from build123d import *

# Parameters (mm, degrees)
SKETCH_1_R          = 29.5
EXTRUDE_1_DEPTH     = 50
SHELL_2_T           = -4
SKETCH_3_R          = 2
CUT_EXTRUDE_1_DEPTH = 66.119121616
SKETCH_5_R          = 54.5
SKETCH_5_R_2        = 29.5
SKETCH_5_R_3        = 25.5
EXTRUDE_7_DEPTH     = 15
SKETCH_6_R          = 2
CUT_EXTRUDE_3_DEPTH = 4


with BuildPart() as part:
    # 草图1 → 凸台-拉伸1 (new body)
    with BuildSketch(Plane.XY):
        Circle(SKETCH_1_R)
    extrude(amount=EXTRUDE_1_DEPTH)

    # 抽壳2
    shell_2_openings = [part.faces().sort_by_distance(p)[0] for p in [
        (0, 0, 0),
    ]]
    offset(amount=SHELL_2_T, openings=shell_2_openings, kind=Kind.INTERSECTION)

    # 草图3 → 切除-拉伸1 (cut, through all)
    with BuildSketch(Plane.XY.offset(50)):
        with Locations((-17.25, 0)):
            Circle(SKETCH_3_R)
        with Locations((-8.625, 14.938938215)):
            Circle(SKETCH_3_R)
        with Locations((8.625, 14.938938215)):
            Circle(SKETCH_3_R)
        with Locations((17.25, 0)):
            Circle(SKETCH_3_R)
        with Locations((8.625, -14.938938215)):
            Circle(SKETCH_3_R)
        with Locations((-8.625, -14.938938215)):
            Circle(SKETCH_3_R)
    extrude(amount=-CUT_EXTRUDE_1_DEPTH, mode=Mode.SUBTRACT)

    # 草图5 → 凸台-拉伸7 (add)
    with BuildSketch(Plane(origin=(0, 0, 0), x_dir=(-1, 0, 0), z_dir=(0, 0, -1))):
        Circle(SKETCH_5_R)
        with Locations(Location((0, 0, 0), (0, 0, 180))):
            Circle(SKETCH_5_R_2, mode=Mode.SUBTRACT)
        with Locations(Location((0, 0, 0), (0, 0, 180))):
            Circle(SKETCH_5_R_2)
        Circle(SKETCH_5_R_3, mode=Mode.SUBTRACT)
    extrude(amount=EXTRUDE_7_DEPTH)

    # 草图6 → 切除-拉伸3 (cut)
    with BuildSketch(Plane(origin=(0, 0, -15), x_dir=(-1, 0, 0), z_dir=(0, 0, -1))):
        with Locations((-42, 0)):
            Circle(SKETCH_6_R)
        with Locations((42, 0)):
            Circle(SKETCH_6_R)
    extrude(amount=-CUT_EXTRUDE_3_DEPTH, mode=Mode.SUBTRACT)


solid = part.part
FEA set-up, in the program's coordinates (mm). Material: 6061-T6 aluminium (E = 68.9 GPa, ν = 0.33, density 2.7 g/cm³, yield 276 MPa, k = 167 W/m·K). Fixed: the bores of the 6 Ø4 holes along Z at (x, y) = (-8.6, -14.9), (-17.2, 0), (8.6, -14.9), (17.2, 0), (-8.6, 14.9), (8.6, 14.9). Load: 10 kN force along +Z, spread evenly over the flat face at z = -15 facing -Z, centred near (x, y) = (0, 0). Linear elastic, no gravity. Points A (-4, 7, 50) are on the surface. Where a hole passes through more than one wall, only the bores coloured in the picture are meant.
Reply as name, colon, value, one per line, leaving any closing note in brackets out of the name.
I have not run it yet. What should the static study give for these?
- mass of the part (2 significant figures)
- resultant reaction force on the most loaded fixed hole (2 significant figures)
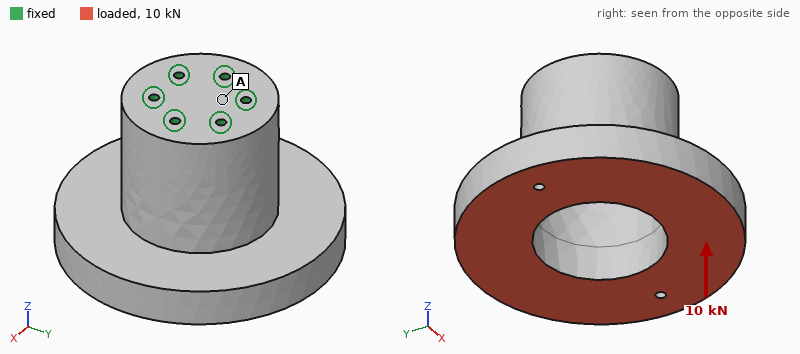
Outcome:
mass of the part: 410 g
resultant reaction force on the most loaded fixed hole: 1.7 kN
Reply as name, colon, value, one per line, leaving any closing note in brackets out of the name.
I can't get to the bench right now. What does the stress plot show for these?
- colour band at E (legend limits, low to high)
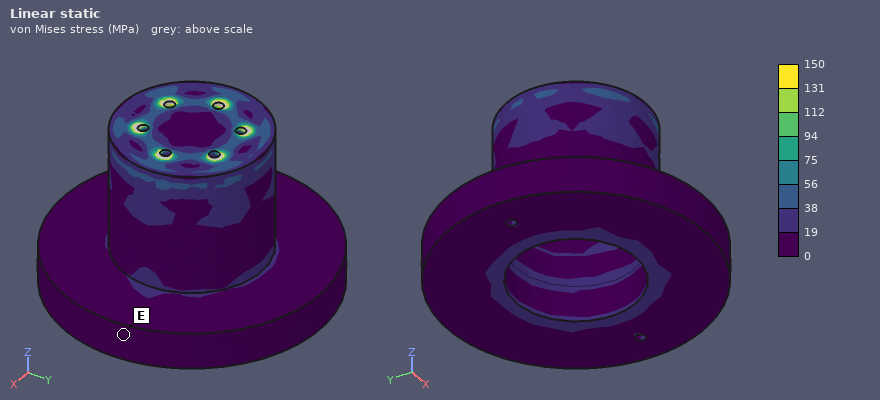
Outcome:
colour band at E: 0 to 19 MPa
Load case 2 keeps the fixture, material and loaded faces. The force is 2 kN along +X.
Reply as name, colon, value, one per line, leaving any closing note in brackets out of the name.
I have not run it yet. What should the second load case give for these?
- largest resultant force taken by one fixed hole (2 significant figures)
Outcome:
largest resultant force taken by one fixed hole: 1.8 kN
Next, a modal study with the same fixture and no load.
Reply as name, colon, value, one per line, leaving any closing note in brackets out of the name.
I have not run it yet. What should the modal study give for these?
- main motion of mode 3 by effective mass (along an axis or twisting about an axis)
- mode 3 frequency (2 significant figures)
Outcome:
main motion of mode 3 by effective mass: twisting about Z
mode 3 frequency: 2900 Hz
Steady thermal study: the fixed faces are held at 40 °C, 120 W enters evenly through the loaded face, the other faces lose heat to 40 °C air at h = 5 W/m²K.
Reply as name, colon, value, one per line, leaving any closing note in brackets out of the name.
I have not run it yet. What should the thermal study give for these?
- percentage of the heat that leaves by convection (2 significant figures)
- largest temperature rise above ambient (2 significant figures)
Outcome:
percentage of the heat that leaves by convection: 6.4 %
largest temperature rise above ambient: 65 K
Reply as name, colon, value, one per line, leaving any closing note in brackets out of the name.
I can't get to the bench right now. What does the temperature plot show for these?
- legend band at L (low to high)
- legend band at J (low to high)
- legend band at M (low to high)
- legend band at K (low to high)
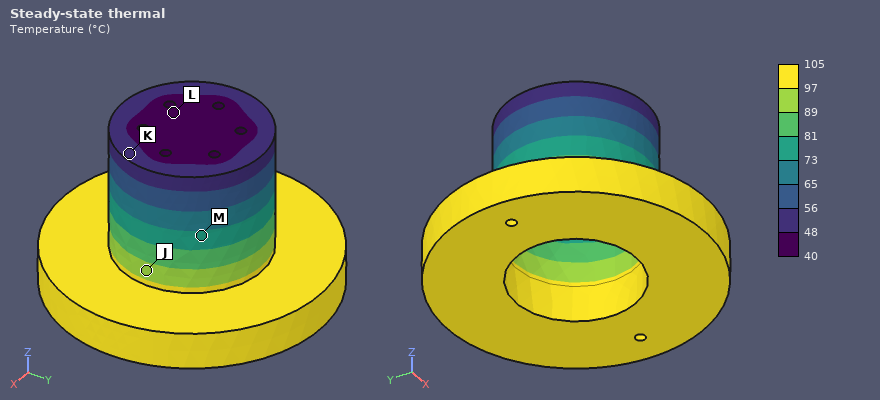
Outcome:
legend band at L: 40 to 48 °C
legend band at J: 89 to 97 °C
legend band at M: 73 to 81 °C
legend band at K: 48 to 56 °C
